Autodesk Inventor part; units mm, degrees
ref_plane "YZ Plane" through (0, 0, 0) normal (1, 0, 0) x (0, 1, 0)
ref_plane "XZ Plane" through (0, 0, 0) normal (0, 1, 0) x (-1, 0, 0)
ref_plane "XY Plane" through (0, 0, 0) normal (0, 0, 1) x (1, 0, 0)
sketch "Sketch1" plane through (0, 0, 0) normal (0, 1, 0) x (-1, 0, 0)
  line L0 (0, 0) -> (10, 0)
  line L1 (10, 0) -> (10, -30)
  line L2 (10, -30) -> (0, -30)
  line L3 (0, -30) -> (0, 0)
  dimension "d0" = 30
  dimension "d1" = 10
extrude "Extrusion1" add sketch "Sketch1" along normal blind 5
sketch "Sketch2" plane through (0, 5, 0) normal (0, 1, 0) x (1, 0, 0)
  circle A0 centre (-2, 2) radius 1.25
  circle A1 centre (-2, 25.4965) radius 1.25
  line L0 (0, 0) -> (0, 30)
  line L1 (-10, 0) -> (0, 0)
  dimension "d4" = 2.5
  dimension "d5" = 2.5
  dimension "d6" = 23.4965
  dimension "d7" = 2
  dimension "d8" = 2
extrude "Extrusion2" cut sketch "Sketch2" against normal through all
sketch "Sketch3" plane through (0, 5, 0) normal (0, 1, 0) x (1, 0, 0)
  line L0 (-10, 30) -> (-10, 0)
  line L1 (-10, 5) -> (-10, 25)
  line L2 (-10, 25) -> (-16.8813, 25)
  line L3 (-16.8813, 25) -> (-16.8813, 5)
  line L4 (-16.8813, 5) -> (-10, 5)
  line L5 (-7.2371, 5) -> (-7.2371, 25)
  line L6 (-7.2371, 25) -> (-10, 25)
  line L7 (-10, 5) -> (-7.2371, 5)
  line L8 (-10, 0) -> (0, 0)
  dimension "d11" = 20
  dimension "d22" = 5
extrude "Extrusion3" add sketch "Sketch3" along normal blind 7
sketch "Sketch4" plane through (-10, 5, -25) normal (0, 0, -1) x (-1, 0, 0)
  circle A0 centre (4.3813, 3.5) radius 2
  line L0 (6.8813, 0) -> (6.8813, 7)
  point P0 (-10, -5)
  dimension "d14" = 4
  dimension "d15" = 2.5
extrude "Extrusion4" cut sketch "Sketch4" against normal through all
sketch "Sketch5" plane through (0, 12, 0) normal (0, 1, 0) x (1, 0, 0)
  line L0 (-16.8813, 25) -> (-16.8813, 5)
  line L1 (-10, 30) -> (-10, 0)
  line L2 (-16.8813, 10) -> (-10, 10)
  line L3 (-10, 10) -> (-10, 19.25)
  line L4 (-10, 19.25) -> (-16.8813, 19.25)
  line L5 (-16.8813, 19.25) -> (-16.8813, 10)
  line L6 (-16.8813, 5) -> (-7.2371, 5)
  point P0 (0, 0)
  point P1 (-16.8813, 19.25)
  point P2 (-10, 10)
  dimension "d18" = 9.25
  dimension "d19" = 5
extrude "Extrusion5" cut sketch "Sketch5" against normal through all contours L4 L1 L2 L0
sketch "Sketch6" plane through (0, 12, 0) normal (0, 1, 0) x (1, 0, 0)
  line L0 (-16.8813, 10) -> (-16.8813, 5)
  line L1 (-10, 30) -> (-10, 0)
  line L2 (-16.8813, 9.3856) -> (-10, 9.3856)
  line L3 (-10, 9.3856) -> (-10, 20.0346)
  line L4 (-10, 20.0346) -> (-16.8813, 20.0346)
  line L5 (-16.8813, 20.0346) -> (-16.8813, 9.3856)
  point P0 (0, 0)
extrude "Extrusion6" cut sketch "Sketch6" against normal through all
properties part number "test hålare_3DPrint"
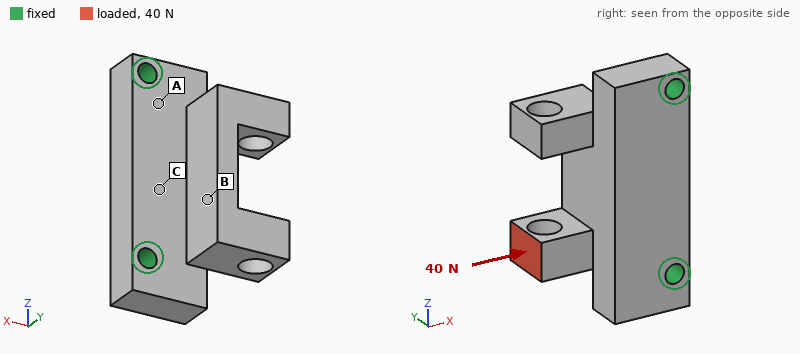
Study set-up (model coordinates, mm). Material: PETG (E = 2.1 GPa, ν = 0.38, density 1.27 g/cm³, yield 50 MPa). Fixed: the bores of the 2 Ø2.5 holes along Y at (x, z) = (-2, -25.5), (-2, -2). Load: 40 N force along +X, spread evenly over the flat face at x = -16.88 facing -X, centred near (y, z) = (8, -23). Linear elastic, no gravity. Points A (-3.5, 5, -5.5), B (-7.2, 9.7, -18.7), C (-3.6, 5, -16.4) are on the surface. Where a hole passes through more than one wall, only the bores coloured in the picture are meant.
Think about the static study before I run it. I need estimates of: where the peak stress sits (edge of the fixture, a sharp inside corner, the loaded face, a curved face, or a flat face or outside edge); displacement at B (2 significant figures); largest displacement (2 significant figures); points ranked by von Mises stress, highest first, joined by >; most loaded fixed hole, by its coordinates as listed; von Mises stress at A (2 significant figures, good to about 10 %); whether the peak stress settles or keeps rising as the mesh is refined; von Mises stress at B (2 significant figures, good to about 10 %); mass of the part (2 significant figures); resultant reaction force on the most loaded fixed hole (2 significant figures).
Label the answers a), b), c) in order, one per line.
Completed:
a) edge of the fixture
b) 0.075 mm
c) 0.20 mm
d) B > A > C
e) (-2, -25.5)
f) 2.1 MPa
g) keeps rising
h) 3.6 MPa
i) 2.8 g
j) 37 N
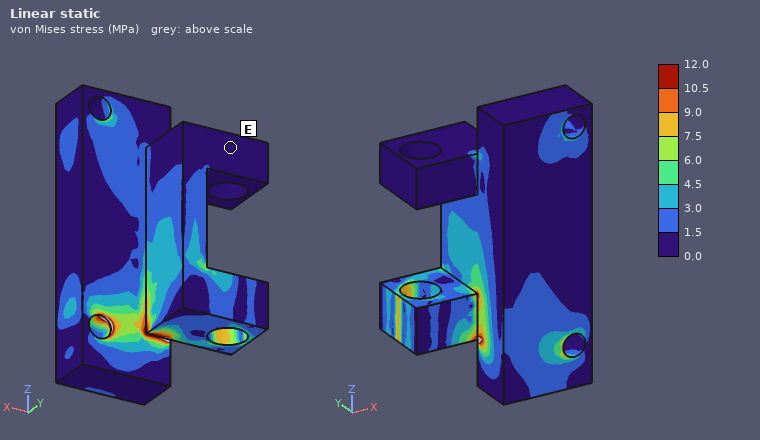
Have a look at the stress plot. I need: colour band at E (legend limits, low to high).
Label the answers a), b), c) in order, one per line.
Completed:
a) 0.0 to 1.5 MPa
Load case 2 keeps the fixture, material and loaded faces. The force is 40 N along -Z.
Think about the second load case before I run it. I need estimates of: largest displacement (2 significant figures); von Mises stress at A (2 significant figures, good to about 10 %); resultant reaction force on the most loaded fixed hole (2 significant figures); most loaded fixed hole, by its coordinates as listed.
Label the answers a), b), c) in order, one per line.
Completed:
a) 0.22 mm
b) 1.7 MPa
c) 41 N
d) (-2, -2)
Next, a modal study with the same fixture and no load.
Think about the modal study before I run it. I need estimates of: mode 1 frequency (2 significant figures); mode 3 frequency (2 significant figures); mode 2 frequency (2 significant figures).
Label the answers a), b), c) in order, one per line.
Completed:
a) 3100 Hz
b) 7100 Hz
c) 4600 Hz
